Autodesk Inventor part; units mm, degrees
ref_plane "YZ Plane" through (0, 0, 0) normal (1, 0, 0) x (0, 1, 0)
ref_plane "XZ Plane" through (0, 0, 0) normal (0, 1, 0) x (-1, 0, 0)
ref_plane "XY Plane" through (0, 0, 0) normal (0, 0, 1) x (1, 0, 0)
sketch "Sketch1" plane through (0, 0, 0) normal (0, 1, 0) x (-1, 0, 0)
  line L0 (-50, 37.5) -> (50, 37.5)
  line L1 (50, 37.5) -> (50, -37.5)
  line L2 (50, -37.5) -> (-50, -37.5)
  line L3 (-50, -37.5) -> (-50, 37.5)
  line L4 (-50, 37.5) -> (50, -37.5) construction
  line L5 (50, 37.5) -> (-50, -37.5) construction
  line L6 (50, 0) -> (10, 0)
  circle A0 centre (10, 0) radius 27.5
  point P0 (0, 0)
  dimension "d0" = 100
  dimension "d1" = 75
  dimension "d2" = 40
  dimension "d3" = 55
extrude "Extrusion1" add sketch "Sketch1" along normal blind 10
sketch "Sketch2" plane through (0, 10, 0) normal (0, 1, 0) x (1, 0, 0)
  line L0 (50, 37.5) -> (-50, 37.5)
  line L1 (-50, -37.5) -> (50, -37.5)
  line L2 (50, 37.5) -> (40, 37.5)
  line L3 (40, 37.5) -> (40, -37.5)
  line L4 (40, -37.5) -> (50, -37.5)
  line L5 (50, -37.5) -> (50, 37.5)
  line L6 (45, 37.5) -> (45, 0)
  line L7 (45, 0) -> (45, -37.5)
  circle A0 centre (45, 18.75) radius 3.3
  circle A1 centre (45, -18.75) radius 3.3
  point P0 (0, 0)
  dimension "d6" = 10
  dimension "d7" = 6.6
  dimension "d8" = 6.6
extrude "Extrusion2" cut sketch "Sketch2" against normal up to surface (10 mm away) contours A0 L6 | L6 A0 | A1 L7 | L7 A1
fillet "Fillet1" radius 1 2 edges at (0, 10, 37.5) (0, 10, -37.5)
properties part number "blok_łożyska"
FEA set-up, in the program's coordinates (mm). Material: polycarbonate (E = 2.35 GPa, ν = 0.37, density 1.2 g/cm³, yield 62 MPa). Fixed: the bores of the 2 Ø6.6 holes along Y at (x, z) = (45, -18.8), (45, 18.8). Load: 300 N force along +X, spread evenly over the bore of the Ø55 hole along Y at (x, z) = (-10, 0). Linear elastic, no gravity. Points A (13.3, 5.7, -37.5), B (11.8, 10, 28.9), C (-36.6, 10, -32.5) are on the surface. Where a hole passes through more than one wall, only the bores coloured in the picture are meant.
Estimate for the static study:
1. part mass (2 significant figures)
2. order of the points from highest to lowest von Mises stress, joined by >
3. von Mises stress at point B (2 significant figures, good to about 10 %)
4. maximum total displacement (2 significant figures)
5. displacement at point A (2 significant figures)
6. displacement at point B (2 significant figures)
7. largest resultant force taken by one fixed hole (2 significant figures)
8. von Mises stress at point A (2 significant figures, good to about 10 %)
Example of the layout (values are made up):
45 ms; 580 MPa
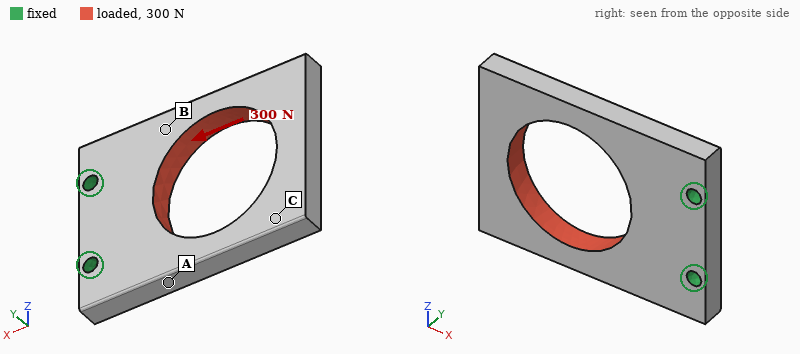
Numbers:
61 g; A > B > C; 0.77 MPa; 65 µm; 23 µm; 18 µm; 160 N; 1.1 MPa
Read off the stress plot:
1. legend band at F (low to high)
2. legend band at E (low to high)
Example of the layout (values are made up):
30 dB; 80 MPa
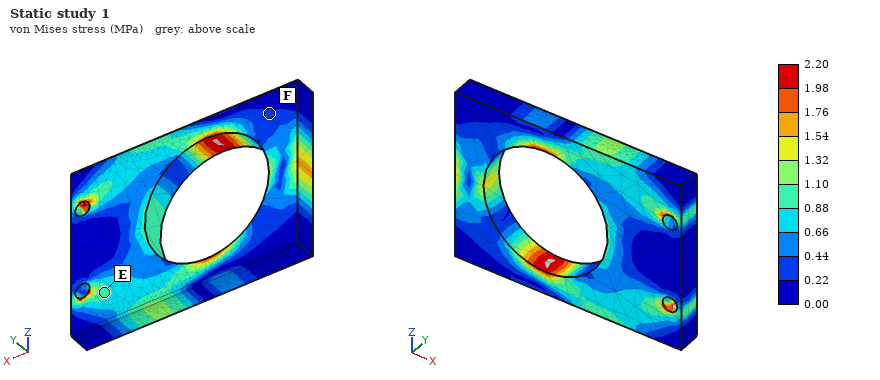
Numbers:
0.22 to 0.44 MPa; 0.88 to 1.10 MPa
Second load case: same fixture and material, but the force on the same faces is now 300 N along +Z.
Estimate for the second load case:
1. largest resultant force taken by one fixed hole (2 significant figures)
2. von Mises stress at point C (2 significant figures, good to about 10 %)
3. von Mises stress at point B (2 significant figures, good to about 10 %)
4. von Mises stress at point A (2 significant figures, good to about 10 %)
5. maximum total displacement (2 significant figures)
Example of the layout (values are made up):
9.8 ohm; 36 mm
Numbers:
400 N; 0.97 MPa; 0.65 MPa; 3.9 MPa; 0.39 mm
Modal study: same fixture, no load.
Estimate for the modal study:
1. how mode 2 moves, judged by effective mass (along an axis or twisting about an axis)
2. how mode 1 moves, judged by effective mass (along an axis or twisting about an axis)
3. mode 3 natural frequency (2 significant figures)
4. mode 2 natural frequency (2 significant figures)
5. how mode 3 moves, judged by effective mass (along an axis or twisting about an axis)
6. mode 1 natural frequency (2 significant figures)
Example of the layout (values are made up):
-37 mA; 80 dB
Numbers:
twisting about X; along Y; 740 Hz; 530 Hz; along Z; 230 Hz
